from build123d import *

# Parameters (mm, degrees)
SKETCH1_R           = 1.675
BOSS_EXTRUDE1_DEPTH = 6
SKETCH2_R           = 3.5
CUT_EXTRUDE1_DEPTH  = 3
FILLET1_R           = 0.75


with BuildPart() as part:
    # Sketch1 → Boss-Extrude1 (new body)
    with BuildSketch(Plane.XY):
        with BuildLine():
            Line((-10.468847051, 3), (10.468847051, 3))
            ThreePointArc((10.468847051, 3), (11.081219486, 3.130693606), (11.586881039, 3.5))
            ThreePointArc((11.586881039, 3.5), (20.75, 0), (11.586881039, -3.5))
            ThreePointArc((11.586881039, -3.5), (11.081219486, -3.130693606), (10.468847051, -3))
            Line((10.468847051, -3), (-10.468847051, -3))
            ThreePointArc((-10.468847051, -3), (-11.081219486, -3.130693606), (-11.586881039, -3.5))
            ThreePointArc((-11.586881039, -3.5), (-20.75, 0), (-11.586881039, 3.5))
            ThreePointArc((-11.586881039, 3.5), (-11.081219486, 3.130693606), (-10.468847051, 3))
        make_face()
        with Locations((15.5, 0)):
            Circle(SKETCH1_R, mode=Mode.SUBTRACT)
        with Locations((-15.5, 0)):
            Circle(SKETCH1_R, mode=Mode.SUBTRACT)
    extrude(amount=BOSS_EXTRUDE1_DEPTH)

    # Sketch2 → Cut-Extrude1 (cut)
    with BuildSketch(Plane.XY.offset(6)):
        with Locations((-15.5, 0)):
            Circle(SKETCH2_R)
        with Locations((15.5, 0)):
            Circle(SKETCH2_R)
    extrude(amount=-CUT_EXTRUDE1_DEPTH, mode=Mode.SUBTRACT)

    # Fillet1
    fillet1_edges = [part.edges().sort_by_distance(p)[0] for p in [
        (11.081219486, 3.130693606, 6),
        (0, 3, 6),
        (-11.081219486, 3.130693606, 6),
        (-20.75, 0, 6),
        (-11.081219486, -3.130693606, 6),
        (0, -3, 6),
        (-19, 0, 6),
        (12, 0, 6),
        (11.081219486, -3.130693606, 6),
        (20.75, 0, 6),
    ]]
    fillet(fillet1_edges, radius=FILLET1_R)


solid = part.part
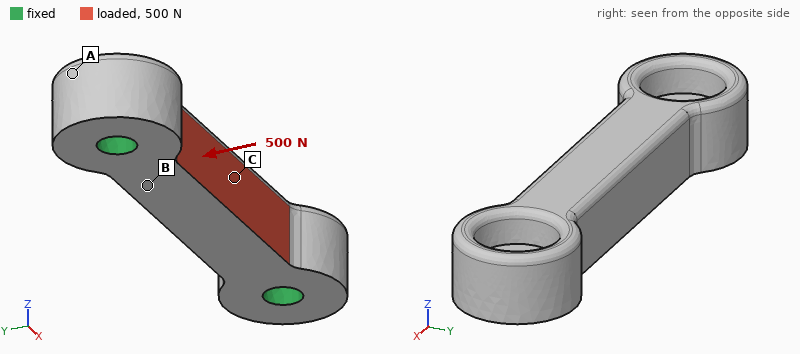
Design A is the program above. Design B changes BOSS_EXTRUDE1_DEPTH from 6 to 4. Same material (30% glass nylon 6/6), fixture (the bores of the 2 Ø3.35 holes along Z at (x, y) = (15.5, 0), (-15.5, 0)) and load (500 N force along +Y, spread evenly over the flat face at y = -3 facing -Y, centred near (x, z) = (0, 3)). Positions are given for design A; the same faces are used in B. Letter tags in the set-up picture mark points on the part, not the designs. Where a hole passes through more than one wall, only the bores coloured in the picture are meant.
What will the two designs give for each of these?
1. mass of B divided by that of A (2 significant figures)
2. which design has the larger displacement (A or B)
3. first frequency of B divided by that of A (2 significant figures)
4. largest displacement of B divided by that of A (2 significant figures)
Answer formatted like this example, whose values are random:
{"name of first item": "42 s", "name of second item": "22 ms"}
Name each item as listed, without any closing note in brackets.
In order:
{"mass of B divided by that of A": "0.70", "which design has the larger displacement": "B", "first frequency of B divided by that of A": "0.85", "largest displacement of B divided by that of A": "1.3"}
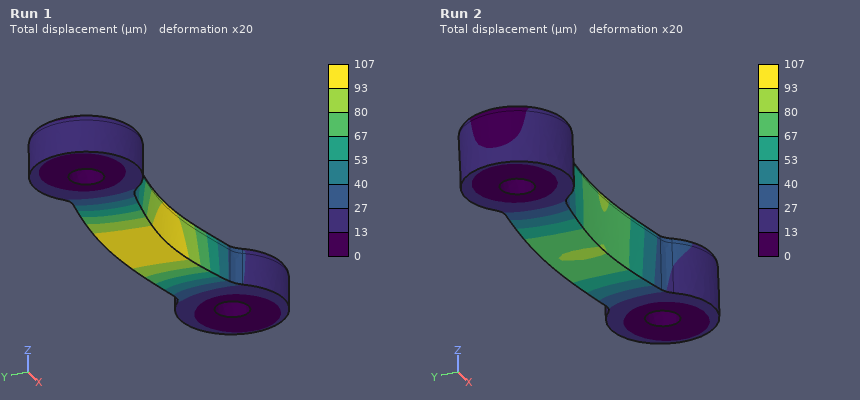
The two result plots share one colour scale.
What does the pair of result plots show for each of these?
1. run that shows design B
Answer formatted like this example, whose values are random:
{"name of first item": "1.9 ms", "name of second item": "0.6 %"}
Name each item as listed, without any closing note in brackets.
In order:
{"run that shows design B": "Run 1"}
